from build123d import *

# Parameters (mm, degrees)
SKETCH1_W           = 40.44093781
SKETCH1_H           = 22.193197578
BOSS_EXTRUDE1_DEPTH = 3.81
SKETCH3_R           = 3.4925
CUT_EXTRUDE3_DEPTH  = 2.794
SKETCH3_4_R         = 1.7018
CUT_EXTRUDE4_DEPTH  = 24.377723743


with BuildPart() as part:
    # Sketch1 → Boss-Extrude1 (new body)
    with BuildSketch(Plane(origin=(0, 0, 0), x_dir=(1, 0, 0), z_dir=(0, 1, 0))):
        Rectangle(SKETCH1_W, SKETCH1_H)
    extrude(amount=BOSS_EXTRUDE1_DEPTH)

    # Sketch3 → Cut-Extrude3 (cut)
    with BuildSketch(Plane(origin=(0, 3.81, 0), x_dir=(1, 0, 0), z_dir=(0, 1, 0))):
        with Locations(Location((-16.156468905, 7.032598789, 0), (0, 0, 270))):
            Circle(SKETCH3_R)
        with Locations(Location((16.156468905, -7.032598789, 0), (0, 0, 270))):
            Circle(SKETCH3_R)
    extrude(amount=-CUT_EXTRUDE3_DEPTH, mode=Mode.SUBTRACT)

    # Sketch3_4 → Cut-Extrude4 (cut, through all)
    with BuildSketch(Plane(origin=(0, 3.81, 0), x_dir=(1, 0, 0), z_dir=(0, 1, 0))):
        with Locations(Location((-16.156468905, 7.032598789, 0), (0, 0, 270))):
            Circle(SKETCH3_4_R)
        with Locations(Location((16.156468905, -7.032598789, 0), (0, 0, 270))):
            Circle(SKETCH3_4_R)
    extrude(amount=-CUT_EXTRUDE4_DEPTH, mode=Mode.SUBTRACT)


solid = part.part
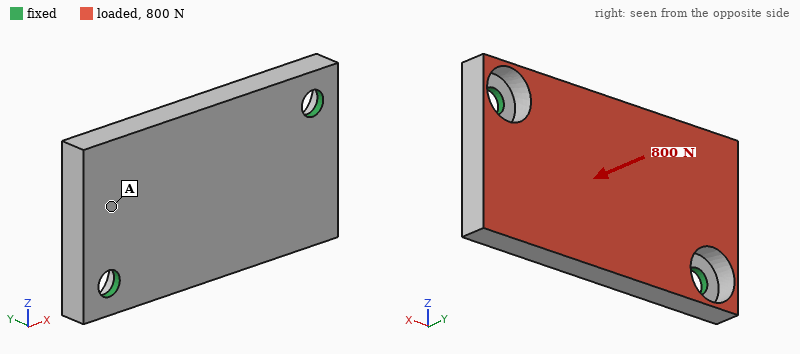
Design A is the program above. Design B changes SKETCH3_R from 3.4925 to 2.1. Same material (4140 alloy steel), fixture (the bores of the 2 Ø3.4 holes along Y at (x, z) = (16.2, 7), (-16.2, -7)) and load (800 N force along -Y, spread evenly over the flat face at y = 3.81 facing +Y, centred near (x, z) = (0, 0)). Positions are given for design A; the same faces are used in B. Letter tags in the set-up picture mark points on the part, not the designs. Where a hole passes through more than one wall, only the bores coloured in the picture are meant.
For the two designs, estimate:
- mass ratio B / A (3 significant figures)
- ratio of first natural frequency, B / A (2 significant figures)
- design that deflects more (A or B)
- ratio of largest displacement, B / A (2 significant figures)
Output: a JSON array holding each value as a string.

["1.04", "1.3", "A", "0.77"]
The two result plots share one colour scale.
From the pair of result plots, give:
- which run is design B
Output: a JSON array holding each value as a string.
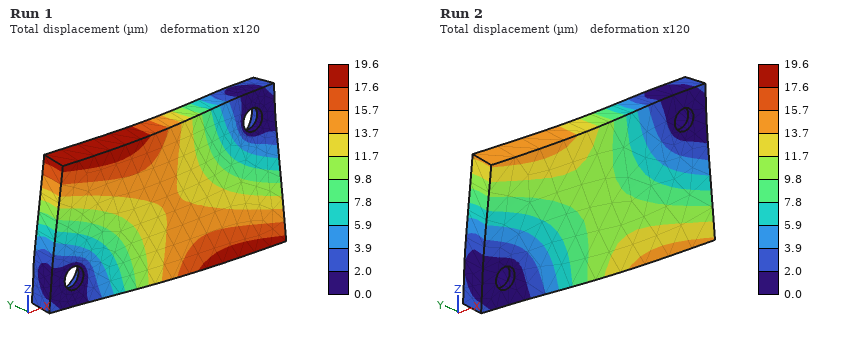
["Run 2"]
